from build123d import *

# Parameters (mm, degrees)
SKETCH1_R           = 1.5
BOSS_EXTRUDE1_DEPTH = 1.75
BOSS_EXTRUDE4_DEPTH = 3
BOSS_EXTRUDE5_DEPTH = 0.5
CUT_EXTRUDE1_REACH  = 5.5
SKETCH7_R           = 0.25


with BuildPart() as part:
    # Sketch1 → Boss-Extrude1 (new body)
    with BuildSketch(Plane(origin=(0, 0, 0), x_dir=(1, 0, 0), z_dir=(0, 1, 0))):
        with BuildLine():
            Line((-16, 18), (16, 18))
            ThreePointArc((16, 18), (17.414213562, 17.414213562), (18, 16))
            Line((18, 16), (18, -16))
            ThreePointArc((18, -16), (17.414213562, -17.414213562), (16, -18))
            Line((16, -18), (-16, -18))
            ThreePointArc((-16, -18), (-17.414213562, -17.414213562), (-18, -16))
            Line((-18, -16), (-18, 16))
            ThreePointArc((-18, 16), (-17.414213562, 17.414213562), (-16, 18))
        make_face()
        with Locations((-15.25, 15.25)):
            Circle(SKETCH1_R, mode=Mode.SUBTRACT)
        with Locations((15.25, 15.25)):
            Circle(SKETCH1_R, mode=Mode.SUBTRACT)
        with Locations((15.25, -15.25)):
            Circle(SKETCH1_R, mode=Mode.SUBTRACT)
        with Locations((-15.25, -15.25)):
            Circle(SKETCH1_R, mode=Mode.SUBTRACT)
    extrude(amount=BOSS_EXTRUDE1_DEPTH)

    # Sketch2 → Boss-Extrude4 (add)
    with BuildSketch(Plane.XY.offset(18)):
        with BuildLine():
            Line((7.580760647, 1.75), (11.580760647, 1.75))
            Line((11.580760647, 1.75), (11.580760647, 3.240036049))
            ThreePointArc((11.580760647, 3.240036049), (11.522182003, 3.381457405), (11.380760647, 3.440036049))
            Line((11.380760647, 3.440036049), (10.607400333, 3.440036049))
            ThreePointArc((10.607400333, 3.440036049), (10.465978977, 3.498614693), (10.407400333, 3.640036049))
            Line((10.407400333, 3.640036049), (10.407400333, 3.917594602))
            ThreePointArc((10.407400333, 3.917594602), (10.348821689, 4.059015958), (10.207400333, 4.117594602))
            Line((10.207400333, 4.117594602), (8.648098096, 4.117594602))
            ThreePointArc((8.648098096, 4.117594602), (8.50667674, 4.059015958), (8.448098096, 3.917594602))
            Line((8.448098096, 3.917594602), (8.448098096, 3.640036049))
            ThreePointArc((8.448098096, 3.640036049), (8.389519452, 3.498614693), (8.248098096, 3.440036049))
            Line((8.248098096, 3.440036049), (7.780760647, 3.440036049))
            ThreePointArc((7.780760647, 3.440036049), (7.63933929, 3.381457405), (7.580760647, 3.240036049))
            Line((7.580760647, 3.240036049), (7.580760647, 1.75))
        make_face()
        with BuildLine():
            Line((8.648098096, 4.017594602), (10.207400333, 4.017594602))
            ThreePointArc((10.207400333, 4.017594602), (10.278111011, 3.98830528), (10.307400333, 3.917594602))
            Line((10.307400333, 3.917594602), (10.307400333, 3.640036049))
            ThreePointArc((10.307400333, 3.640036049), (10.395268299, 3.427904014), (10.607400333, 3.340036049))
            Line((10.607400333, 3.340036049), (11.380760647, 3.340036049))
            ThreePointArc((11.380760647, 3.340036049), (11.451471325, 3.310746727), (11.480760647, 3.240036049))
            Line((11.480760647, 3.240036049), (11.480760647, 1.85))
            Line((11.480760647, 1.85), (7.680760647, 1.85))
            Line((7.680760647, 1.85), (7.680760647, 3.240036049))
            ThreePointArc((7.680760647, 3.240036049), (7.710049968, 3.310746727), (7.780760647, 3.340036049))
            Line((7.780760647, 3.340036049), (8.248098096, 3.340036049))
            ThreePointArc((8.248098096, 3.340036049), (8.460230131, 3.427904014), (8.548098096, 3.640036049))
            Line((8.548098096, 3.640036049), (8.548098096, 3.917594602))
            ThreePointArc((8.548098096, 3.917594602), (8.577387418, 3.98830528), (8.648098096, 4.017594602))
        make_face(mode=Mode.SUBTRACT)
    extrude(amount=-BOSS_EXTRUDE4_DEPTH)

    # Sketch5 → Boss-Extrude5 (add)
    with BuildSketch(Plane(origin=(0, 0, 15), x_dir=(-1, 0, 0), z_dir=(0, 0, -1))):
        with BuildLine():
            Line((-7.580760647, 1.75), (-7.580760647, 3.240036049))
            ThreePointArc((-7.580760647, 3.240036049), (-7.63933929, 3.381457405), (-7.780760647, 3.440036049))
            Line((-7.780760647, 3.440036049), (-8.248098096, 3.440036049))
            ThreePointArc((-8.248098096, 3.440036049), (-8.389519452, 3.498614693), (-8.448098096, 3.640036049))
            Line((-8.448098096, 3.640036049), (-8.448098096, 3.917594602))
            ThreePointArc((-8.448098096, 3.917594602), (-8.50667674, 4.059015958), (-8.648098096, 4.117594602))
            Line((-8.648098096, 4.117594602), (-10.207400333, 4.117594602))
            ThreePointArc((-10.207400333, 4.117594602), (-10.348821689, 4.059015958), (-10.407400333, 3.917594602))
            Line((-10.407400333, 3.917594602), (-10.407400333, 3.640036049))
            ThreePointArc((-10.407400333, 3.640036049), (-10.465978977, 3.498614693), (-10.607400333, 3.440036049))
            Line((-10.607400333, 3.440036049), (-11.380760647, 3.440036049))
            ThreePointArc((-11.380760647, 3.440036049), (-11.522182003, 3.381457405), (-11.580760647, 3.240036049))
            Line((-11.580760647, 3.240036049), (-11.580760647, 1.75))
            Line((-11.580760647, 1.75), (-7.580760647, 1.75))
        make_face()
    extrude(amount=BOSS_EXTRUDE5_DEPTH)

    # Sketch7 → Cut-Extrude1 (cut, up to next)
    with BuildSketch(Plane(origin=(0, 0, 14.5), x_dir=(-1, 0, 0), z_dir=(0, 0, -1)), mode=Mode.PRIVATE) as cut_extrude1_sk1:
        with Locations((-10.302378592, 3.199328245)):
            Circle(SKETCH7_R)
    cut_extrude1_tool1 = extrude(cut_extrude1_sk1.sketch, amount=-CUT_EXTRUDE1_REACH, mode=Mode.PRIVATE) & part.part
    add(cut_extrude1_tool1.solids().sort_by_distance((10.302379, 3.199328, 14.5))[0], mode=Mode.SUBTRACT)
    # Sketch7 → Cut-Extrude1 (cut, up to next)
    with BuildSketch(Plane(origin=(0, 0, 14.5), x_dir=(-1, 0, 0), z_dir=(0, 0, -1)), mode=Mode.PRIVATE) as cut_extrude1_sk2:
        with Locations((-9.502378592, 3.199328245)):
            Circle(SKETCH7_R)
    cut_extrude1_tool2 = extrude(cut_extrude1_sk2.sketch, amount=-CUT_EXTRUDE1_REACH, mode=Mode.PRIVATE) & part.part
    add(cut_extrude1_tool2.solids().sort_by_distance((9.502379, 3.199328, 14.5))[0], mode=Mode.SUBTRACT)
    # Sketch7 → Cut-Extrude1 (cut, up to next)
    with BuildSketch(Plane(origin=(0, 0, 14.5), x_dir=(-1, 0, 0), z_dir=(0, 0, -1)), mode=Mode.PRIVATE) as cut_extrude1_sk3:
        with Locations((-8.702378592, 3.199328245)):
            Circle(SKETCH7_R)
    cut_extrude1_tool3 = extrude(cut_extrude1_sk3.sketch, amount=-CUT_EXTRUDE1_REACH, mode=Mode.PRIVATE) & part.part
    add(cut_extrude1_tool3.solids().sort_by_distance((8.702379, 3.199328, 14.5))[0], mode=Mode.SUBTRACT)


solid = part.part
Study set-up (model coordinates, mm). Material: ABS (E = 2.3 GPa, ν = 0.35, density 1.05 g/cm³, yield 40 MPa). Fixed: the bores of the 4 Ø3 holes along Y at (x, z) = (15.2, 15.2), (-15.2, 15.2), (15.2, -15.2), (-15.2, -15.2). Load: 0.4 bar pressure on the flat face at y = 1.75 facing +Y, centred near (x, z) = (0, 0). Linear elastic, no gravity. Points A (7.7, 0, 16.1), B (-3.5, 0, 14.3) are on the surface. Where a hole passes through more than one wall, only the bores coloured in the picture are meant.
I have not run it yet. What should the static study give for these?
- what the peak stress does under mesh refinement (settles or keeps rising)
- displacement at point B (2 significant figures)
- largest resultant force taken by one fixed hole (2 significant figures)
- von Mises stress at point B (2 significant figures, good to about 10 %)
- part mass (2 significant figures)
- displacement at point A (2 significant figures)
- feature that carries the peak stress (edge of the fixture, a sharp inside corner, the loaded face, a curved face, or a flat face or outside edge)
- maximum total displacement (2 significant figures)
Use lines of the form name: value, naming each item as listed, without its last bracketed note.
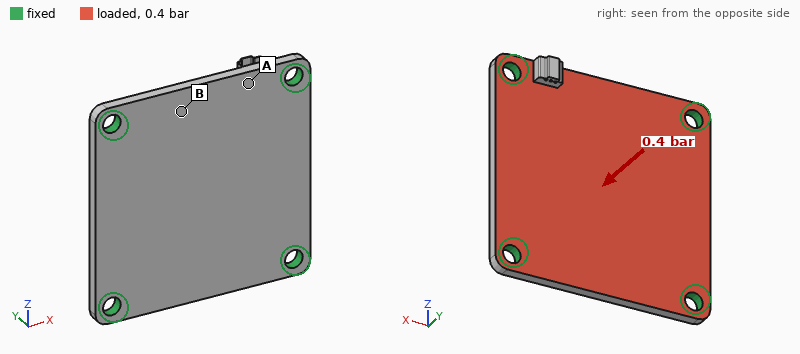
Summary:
what the peak stress does under mesh refinement: keeps rising
displacement at point B: 0.095 mm
largest resultant force taken by one fixed hole: 13 N
von Mises stress at point B: 3.0 MPa
part mass: 2.3 g
displacement at point A: 0.047 mm
feature that carries the peak stress: edge of the fixture
maximum total displacement: 0.19 mm
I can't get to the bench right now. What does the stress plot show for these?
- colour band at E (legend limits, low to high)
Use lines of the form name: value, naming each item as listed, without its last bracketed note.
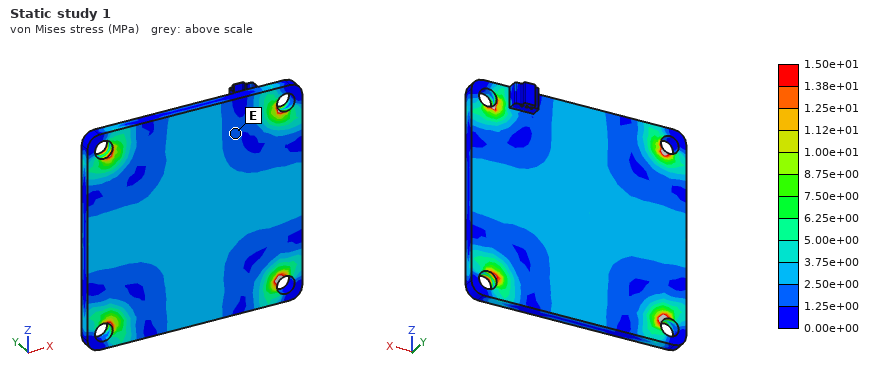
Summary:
colour band at E: 1.25e+00 to 2.50e+00 MPa
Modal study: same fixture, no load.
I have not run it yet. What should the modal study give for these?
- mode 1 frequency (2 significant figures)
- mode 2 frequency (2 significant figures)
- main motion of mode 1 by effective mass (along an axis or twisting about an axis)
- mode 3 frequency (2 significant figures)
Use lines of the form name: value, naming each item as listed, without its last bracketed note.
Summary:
mode 1 frequency: 2100 Hz
mode 2 frequency: 3500 Hz
main motion of mode 1 by effective mass: along Y
mode 3 frequency: 3500 Hz
